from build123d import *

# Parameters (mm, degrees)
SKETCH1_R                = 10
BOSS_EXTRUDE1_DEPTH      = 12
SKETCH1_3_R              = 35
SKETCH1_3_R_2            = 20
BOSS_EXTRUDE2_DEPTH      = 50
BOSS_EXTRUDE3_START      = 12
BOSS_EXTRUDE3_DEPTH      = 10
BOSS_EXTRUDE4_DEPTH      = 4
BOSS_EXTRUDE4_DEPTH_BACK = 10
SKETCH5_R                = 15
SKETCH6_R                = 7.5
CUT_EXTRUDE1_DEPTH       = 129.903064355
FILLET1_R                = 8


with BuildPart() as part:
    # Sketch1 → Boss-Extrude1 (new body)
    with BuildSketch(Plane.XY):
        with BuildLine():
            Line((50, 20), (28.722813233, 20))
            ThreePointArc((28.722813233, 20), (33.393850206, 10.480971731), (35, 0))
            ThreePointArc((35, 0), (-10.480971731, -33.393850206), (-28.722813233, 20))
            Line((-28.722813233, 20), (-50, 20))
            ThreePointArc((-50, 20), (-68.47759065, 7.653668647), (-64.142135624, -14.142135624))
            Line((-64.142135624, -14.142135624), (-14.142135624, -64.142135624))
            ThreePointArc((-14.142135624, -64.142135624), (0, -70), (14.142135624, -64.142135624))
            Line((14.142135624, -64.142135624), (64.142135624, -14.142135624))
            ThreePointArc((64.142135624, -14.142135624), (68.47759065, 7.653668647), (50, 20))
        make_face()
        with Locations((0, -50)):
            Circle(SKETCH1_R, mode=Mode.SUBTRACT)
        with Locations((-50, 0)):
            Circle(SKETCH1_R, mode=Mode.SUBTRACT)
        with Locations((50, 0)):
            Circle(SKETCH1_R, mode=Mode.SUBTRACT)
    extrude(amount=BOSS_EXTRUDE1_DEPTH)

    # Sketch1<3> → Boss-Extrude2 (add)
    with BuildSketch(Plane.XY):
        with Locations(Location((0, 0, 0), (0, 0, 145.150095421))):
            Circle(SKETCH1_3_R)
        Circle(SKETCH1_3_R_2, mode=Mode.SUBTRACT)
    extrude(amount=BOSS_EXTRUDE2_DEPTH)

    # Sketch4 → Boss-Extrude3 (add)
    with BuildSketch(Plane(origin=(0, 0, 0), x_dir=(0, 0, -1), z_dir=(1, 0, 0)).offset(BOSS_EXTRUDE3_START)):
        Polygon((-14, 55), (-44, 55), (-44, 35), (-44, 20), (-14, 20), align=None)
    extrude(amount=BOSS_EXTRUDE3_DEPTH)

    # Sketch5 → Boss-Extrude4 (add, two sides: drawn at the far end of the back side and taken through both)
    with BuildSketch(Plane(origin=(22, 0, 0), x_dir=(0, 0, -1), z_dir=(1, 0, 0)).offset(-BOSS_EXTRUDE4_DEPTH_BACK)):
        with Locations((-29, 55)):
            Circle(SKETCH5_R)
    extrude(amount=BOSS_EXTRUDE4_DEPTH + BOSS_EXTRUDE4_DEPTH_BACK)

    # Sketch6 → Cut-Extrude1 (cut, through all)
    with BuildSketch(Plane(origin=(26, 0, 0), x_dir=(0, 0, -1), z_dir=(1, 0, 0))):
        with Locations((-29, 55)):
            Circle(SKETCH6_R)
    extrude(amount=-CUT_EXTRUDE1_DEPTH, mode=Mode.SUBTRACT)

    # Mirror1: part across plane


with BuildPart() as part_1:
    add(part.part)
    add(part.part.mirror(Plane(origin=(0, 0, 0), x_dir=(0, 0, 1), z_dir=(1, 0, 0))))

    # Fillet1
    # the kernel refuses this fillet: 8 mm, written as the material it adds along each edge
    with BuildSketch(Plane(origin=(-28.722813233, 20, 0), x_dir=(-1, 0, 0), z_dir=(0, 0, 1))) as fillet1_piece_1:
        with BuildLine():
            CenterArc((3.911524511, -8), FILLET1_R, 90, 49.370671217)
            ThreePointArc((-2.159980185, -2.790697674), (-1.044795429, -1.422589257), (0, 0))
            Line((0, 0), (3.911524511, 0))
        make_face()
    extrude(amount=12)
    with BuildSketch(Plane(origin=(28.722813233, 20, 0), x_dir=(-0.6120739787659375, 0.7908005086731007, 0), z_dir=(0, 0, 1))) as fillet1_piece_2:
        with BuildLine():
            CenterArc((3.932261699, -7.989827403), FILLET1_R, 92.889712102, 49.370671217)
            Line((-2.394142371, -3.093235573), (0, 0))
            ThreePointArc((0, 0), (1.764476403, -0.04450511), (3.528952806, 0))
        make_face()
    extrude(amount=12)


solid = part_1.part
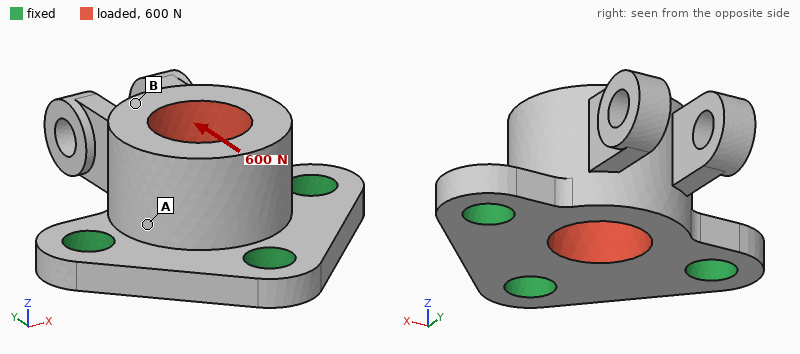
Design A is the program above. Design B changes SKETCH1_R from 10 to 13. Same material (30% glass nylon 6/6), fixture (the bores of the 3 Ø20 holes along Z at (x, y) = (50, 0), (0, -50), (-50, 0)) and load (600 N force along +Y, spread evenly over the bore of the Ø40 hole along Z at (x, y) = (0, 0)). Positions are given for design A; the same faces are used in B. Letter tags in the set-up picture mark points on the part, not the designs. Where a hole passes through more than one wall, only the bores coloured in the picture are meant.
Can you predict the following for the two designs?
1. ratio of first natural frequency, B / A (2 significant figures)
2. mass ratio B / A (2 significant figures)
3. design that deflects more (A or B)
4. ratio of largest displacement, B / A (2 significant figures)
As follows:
1.1
0.96
A
0.80
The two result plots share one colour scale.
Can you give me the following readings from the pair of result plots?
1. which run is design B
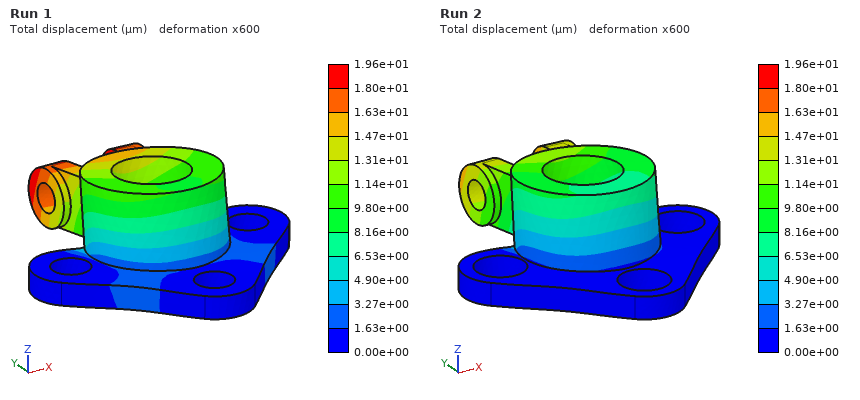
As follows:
Run 2
